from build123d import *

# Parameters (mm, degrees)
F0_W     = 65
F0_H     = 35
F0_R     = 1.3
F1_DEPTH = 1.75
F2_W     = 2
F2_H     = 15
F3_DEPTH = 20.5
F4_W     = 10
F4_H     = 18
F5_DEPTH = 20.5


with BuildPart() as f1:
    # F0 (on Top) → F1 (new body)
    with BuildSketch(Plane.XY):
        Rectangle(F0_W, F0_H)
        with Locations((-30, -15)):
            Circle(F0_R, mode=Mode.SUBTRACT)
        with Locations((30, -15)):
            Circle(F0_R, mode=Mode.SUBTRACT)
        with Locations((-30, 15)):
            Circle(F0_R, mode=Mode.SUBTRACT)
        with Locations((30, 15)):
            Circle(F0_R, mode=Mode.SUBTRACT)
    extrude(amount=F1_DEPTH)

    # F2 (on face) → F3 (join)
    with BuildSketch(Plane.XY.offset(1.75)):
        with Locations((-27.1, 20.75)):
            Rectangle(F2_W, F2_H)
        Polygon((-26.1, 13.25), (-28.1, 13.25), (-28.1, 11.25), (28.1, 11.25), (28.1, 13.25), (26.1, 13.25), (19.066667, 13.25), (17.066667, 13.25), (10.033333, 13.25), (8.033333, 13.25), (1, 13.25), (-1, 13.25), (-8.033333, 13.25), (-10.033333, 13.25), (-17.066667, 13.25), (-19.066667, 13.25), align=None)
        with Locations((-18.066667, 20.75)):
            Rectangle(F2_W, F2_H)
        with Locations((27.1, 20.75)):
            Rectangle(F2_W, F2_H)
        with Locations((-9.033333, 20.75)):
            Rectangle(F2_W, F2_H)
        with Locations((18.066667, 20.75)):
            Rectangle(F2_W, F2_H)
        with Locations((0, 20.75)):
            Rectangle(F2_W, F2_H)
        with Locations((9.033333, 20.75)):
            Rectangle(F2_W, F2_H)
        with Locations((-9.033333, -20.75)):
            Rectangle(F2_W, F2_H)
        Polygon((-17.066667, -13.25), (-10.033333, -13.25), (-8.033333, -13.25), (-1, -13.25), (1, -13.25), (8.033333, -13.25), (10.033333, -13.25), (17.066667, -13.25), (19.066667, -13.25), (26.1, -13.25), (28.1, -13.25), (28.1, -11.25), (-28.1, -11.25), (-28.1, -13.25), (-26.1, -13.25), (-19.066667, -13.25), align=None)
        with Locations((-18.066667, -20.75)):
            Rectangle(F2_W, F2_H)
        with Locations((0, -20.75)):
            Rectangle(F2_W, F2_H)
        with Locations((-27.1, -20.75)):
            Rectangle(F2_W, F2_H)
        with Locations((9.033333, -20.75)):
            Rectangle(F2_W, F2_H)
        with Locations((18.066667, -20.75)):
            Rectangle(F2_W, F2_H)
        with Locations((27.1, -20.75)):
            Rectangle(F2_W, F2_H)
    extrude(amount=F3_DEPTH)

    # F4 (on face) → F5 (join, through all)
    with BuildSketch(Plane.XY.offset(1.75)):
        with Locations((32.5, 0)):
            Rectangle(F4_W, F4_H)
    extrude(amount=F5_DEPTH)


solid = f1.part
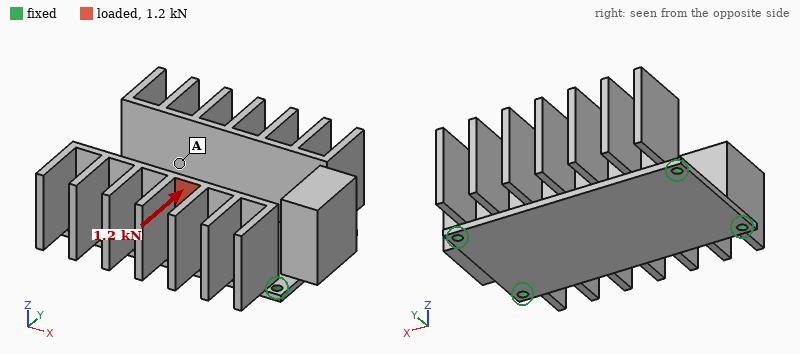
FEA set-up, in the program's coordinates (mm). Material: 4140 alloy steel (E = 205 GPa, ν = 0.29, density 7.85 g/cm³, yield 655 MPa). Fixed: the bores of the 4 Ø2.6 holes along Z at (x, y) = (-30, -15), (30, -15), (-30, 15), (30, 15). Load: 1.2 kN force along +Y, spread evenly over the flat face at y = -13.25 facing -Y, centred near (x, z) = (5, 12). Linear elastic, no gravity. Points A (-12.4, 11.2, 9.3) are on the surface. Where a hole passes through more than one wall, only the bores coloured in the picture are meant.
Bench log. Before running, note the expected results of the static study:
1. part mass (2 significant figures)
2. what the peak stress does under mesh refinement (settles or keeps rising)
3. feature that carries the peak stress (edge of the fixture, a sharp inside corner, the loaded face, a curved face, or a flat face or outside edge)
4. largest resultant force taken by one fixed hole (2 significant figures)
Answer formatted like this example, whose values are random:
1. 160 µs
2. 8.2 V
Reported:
1. 160 g
2. keeps rising
3. edge of the fixture
4. 580 N
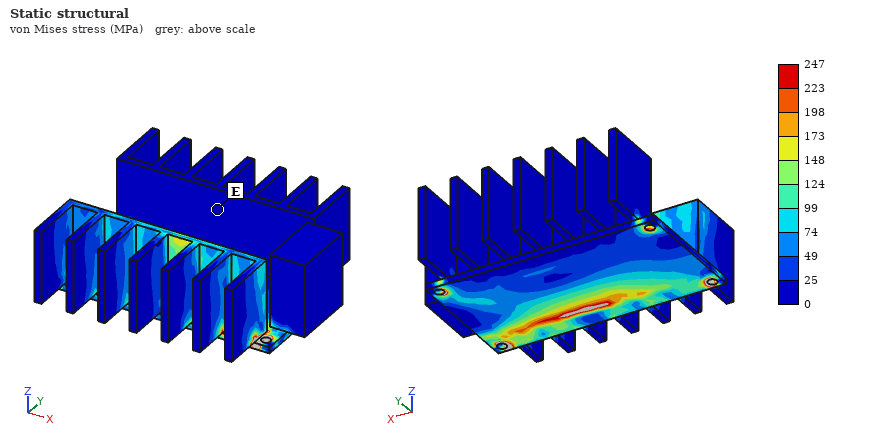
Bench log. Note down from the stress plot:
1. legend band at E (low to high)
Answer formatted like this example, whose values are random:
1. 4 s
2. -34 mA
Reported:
1. 0 to 25 MPa
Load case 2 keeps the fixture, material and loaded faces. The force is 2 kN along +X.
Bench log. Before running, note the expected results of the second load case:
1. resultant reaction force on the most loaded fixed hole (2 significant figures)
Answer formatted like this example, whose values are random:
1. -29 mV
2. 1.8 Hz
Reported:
1. 860 N
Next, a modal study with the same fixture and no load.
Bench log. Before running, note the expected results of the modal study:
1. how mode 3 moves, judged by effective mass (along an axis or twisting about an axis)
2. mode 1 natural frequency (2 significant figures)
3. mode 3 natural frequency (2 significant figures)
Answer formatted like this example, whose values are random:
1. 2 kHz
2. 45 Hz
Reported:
1. along Y
2. 1800 Hz
3. 2500 Hz
